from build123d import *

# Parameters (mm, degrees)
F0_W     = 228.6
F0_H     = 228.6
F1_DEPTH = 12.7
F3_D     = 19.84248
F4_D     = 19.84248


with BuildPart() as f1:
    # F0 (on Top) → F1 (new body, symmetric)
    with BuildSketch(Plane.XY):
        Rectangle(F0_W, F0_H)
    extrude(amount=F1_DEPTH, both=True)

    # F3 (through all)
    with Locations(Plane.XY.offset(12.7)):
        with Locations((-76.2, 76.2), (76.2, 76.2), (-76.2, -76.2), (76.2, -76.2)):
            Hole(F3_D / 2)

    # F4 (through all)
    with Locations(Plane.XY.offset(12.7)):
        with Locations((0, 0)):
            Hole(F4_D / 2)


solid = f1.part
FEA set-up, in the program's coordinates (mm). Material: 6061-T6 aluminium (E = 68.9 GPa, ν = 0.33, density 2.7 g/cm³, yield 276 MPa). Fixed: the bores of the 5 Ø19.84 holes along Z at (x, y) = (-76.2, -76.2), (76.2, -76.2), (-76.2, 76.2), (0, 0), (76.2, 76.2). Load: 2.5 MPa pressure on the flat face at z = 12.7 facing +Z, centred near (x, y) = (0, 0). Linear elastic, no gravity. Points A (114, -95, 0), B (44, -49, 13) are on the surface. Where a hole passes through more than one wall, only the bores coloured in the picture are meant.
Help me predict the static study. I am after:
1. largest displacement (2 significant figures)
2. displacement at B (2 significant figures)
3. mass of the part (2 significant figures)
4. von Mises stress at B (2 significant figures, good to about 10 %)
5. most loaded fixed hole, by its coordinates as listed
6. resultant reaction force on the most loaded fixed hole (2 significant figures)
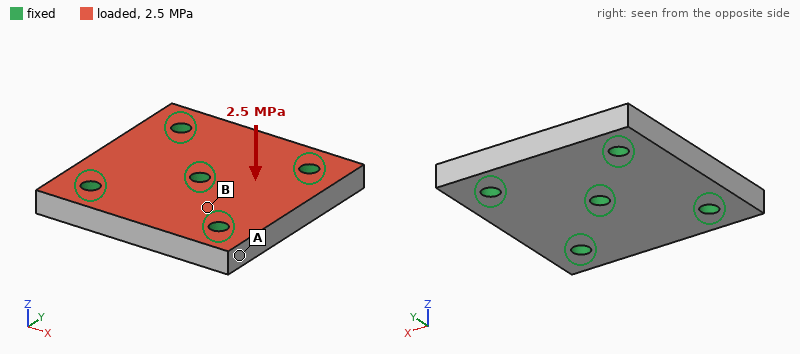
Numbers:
47 µm
18 µm
3.5 kg
17 MPa
(0, 0)
28 kN
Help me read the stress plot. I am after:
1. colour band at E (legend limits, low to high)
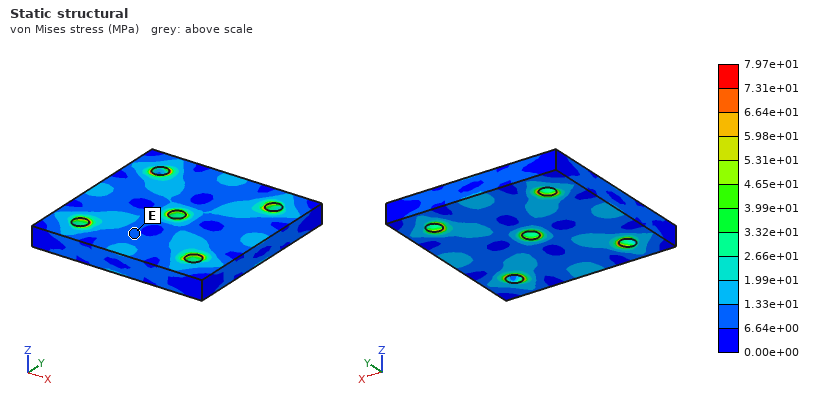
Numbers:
6.64e+00 to 1.33e+01 MPa
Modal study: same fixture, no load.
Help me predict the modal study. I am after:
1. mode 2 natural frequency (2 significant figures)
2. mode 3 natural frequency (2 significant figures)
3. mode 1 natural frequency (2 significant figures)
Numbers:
5400 Hz
5400 Hz
5100 Hz
